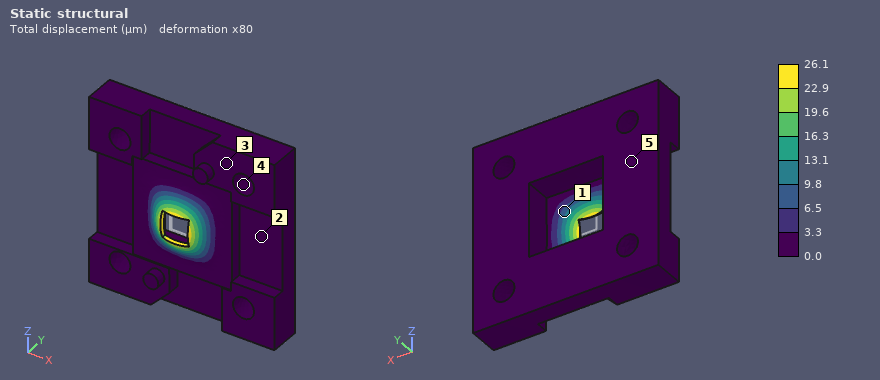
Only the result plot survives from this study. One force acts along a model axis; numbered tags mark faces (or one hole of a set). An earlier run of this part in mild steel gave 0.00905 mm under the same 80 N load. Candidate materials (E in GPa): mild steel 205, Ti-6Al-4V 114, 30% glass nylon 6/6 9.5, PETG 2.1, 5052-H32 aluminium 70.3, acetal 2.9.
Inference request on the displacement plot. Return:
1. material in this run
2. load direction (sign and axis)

5052-H32 aluminium
-Y
